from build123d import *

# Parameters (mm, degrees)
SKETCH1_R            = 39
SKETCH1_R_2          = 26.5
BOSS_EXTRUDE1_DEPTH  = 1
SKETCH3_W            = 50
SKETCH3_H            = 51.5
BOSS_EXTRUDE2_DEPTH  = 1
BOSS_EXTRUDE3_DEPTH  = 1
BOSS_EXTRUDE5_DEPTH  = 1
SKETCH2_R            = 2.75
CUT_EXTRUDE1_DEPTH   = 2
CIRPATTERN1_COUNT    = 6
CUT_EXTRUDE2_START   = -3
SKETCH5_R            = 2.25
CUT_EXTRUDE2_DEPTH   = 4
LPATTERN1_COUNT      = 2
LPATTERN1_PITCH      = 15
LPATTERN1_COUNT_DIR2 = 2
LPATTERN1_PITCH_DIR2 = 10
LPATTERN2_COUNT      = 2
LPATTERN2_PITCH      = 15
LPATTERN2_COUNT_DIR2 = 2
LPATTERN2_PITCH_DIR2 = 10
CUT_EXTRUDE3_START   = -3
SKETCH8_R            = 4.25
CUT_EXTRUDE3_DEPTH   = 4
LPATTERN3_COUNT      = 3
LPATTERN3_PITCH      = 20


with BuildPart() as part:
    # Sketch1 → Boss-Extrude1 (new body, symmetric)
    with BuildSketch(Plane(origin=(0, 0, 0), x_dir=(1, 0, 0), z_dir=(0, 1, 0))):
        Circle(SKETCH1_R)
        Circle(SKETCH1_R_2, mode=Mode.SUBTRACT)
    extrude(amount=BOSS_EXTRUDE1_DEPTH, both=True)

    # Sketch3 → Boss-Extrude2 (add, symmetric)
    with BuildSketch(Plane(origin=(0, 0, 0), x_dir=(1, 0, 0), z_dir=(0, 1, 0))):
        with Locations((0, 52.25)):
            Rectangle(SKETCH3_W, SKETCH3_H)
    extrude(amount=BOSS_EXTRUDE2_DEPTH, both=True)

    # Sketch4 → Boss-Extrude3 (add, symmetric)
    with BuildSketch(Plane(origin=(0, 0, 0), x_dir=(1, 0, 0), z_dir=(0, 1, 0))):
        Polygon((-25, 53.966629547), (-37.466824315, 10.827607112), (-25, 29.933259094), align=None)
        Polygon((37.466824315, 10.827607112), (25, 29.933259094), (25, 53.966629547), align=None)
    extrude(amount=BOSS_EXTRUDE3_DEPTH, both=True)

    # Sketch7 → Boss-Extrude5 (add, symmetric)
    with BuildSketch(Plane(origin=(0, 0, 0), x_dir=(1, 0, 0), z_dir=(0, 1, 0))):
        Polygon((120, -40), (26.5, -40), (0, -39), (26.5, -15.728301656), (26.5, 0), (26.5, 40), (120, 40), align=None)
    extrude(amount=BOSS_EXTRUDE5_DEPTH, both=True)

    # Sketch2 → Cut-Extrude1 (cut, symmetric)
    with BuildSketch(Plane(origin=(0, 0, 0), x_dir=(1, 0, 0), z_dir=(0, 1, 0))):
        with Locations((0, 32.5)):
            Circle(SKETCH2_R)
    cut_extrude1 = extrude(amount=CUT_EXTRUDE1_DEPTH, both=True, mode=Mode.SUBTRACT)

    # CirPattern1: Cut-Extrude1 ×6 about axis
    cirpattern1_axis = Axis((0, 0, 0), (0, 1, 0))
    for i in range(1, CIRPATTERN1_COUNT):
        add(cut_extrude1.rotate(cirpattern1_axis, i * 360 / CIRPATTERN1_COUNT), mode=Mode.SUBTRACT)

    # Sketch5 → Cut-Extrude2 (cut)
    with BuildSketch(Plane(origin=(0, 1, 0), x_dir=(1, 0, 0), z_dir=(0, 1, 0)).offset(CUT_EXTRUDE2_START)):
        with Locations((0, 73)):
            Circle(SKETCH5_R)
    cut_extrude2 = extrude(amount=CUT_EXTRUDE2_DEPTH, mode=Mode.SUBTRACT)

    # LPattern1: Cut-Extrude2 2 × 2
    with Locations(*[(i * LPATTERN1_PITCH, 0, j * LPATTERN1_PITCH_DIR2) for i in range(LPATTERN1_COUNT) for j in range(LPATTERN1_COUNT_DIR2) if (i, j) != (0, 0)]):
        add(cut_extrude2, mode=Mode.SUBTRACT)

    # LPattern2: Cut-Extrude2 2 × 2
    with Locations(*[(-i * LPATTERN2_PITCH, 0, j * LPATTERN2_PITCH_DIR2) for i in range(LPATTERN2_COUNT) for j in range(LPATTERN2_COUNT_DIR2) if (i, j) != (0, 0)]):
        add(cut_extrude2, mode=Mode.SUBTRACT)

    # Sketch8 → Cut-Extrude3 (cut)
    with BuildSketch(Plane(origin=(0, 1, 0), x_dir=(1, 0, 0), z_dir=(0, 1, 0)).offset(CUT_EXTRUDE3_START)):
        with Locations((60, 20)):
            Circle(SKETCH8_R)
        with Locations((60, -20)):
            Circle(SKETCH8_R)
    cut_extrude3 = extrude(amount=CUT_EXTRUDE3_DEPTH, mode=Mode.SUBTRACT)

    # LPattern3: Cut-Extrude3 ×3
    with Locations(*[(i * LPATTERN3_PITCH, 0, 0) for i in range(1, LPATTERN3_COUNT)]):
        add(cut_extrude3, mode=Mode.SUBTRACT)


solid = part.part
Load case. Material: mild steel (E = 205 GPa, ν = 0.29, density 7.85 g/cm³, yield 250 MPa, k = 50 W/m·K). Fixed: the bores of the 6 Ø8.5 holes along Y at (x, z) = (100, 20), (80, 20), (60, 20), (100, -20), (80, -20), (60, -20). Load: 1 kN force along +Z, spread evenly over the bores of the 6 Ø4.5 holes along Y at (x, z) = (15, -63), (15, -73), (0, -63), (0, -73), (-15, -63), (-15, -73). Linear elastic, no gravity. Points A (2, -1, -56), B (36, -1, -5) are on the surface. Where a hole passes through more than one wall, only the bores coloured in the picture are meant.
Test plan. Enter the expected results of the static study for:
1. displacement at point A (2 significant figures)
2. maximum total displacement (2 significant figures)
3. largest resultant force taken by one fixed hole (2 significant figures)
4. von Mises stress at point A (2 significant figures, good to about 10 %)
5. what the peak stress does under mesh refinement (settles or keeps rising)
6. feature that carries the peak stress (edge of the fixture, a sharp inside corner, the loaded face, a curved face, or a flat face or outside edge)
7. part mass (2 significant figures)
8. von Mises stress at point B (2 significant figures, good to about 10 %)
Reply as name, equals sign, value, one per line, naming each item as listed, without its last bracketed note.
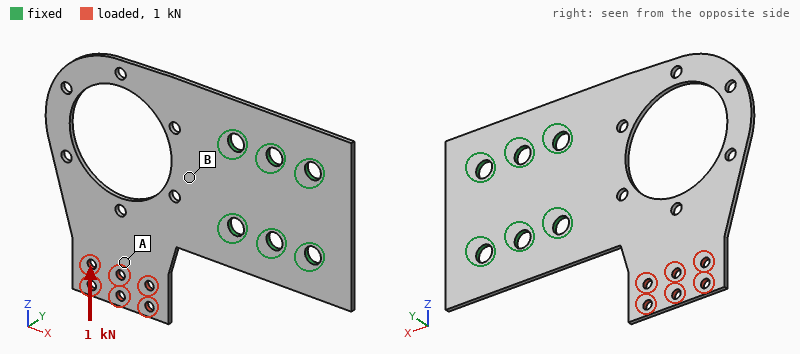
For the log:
displacement at point A = 39 µm
maximum total displacement = 65 µm
largest resultant force taken by one fixed hole = 1.0 kN
von Mises stress at point A = 8.4 MPa
what the peak stress does under mesh refinement = keeps rising
feature that carries the peak stress = a sharp inside corner
part mass = 180 g
von Mises stress at point B = 30 MPa
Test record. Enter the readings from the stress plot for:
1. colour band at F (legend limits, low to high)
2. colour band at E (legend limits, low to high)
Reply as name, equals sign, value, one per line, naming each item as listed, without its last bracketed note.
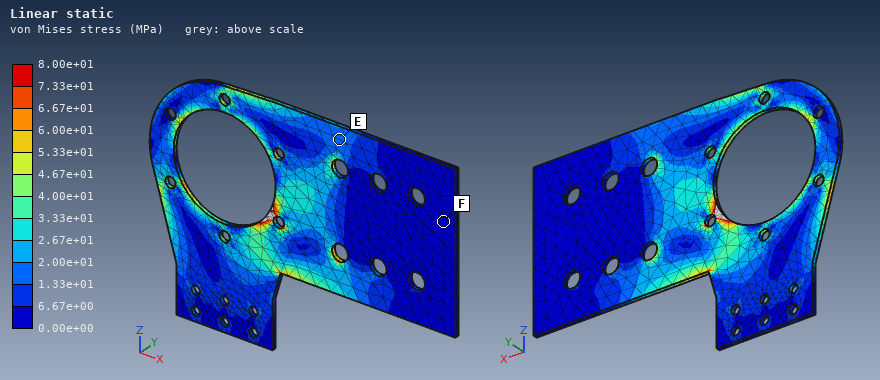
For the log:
colour band at F = 0.00e+00 to 6.67e+00 MPa
colour band at E = 1.33e+01 to 2.00e+01 MPa
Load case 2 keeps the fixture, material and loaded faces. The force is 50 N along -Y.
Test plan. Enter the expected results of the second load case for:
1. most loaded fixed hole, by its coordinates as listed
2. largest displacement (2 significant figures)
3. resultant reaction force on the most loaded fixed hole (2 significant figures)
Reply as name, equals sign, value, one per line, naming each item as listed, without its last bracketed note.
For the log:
most loaded fixed hole, by its coordinates as listed = (60, -20)
largest displacement = 1.9 mm
resultant reaction force on the most loaded fixed hole = 110 N
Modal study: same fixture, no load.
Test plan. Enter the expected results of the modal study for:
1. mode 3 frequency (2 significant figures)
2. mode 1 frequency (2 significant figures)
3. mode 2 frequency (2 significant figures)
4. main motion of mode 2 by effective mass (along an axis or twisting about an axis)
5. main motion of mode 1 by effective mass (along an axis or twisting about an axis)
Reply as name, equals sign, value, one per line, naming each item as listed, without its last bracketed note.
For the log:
mode 3 frequency = 750 Hz
mode 1 frequency = 160 Hz
mode 2 frequency = 320 Hz
main motion of mode 2 by effective mass = twisting about X
main motion of mode 1 by effective mass = along Y
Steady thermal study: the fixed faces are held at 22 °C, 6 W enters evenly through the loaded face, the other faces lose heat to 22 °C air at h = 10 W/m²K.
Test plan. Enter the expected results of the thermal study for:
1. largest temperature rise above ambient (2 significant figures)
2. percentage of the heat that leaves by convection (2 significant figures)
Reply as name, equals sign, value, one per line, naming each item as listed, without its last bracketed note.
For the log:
largest temperature rise above ambient = 68 K
percentage of the heat that leaves by convection = 62 %
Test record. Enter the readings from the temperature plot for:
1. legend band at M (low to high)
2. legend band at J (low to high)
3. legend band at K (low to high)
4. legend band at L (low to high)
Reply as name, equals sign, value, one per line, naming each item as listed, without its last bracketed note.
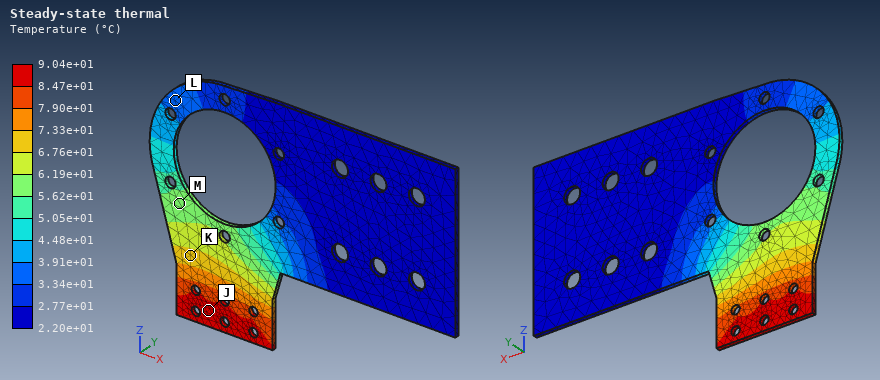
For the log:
legend band at M = 5.62e+01 to 6.19e+01 °C
legend band at J = 8.47e+01 to 9.04e+01 °C
legend band at K = 6.76e+01 to 7.33e+01 °C
legend band at L = 3.34e+01 to 3.91e+01 °C
